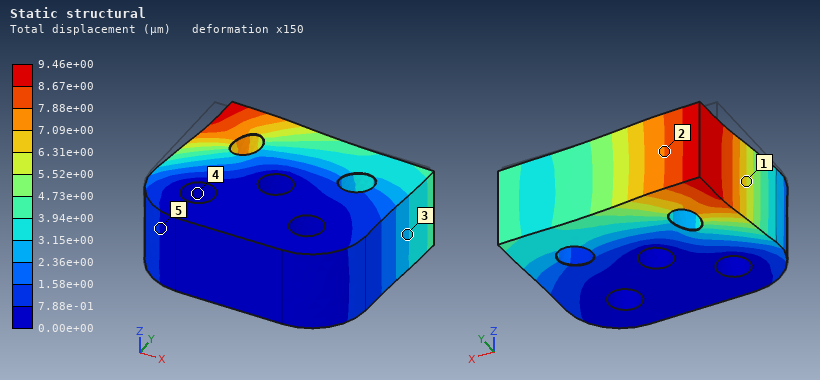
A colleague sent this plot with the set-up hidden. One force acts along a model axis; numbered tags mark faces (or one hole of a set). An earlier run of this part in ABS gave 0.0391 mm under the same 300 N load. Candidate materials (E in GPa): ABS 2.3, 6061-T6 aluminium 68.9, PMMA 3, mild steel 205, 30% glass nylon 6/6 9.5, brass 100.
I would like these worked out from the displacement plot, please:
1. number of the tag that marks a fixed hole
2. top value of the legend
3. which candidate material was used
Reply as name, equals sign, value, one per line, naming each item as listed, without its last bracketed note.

number of the tag that marks a fixed hole = 4
top value of the legend = 9.46e+00 µm
which candidate material was used = 30% glass nylon 6/6
